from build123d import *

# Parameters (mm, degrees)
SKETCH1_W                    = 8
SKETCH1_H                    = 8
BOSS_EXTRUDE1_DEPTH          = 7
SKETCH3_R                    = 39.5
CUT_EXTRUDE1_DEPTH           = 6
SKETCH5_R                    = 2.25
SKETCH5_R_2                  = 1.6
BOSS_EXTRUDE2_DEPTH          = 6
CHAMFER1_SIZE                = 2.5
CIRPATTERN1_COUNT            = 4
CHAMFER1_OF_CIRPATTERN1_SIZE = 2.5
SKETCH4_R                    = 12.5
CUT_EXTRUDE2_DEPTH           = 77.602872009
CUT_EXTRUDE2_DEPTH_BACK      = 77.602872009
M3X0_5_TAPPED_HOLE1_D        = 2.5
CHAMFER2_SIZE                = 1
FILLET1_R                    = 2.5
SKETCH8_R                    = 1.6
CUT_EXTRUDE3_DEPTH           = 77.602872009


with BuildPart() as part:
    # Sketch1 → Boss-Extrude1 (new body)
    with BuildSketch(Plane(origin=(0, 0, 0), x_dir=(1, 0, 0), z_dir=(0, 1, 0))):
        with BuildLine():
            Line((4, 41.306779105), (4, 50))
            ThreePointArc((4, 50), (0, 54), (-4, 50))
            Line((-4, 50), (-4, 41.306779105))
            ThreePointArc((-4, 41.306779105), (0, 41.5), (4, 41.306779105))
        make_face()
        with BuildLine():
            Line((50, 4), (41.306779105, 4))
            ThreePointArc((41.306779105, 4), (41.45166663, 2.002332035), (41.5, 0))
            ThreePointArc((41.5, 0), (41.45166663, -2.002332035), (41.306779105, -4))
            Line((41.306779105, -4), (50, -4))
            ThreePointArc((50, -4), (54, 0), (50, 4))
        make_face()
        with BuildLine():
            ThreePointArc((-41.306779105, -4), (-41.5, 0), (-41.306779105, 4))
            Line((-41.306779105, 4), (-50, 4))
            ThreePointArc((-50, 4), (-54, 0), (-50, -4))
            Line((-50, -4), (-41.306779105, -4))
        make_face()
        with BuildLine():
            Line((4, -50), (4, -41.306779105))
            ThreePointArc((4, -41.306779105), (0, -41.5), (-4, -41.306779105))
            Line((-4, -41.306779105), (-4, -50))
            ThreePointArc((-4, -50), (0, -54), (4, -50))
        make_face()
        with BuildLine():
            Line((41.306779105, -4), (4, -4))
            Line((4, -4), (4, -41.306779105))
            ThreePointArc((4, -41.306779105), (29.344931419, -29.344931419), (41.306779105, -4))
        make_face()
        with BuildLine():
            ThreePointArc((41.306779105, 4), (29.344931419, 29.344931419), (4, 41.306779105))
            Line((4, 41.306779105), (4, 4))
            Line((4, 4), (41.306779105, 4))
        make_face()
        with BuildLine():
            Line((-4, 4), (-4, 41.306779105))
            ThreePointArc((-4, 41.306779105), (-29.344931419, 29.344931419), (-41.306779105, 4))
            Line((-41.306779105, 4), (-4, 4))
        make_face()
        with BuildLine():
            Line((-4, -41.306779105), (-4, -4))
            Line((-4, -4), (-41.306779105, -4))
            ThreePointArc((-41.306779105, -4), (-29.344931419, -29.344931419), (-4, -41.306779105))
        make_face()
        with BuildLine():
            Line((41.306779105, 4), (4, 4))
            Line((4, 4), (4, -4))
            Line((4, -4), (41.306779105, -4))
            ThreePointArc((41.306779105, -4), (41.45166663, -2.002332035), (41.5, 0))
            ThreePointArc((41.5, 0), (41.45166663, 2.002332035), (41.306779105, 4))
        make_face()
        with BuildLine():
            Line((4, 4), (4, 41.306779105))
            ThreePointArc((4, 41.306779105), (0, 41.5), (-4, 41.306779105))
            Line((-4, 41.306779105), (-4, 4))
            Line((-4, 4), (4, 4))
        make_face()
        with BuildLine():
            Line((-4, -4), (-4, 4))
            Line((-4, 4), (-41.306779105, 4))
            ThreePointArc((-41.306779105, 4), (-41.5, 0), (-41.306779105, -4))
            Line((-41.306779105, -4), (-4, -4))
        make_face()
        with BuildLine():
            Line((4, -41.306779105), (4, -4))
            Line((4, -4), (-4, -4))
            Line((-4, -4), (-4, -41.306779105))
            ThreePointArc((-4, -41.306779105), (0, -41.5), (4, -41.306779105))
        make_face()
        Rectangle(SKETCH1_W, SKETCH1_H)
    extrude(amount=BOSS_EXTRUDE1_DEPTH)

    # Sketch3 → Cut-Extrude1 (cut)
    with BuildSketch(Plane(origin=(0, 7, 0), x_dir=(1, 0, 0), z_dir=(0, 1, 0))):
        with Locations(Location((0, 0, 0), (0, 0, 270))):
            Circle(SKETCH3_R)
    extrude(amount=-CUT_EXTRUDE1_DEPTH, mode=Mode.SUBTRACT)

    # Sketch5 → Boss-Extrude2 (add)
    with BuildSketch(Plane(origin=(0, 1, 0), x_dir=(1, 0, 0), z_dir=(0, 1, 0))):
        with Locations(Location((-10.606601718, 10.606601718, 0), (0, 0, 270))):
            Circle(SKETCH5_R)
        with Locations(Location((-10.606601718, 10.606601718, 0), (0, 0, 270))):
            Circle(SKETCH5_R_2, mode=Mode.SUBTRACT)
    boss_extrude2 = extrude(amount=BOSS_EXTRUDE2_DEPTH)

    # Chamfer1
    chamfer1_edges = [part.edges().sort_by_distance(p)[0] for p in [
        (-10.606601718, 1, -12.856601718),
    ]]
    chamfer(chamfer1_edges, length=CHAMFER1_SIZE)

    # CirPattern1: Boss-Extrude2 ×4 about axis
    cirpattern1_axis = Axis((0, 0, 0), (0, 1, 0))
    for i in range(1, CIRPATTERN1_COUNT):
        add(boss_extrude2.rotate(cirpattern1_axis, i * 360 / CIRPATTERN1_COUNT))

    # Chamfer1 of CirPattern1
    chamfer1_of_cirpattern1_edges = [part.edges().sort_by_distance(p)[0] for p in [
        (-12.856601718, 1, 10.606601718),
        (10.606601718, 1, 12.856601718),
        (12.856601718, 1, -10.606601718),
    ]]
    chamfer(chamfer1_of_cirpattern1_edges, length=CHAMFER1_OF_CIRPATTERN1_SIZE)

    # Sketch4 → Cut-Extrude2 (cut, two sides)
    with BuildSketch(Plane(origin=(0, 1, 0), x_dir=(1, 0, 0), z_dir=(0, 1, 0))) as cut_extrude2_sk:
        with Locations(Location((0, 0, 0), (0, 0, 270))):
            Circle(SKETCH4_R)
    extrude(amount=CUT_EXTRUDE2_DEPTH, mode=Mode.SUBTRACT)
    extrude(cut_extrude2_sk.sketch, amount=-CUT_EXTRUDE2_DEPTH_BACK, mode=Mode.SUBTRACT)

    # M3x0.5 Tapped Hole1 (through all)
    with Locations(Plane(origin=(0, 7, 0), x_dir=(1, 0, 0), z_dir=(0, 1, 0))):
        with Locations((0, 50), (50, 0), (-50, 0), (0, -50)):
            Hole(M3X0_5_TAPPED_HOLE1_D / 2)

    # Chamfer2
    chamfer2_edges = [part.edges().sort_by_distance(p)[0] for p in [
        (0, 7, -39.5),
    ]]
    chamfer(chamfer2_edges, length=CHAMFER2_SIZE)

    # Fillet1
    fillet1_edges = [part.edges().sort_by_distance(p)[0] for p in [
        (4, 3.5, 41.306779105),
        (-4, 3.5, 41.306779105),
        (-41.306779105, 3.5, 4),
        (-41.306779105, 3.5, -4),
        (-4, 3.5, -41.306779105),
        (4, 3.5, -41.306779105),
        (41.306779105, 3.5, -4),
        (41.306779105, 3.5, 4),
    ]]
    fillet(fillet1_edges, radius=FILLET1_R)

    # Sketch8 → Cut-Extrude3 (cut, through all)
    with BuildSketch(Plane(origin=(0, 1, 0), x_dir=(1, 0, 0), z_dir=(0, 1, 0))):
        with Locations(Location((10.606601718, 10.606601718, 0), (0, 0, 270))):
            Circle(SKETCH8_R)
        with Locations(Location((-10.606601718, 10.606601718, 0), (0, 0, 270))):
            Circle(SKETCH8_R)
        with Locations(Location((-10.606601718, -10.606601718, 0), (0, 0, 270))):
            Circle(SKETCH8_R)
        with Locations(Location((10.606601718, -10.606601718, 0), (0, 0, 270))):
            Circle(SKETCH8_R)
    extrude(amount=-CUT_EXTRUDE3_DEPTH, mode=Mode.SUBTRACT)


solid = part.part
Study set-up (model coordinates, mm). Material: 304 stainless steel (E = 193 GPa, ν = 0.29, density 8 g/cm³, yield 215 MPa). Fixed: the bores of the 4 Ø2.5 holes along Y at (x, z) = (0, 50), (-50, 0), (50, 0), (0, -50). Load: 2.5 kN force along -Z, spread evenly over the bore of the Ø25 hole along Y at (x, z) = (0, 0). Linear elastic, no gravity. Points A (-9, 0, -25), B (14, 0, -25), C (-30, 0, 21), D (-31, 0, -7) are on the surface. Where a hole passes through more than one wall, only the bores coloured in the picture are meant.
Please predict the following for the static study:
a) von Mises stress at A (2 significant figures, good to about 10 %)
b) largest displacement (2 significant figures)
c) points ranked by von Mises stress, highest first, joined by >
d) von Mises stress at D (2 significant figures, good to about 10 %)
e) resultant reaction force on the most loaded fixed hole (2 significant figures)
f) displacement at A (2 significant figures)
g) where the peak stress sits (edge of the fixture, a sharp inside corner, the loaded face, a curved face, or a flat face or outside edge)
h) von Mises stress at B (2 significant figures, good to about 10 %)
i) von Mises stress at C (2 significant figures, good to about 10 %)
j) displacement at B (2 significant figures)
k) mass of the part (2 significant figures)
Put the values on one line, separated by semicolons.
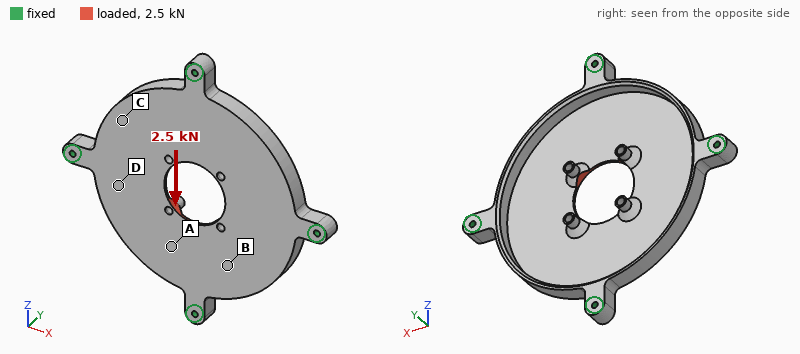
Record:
35 MPa; 24 µm; A > B > C > D; 6.5 MPa; 880 N; 17 µm; a curved face; 26 MPa; 13 MPa; 16 µm; 86 g
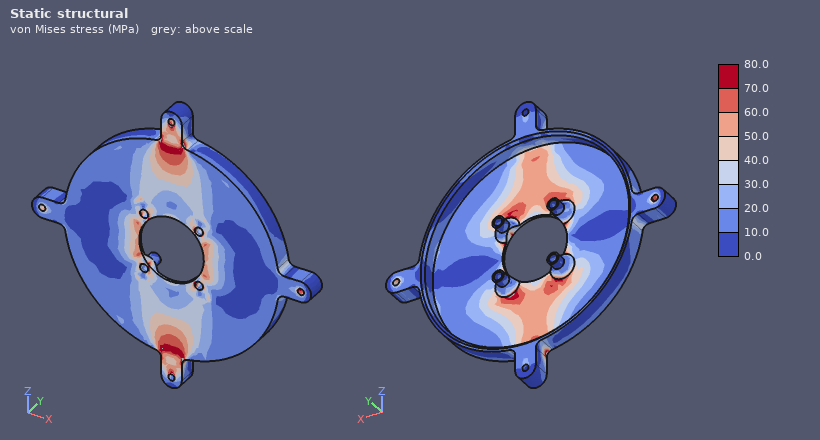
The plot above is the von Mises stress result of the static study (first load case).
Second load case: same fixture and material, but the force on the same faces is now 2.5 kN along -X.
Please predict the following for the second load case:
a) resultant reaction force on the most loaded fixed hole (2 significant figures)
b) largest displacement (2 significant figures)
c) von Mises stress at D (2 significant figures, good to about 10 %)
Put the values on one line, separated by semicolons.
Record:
880 N; 24 µm; 45 MPa
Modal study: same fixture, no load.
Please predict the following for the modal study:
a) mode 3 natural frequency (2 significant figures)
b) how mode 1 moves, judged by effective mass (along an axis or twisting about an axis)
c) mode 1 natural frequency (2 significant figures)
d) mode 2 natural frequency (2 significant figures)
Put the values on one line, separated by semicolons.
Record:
2700 Hz; along Y; 1500 Hz; 2700 Hz
